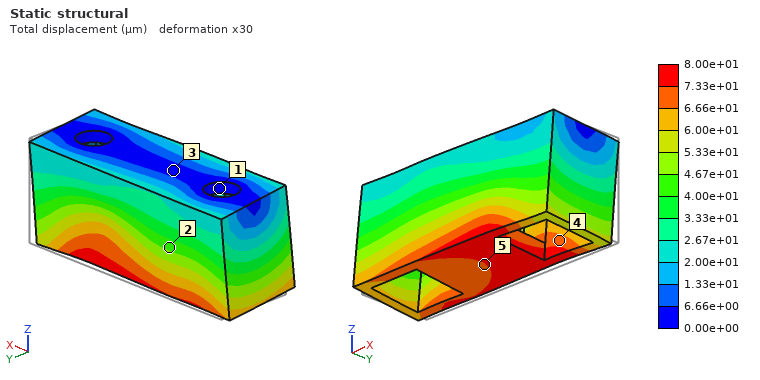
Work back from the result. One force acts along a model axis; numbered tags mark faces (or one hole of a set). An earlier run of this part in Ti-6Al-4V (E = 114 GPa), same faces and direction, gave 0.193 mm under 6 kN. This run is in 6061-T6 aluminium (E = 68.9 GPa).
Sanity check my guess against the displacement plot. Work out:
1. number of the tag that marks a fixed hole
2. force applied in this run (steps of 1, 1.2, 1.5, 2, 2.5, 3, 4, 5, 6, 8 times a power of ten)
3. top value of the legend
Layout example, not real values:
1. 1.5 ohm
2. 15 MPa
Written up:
1. 1
2. 1.5 kN
3. 8.00e+01 µm
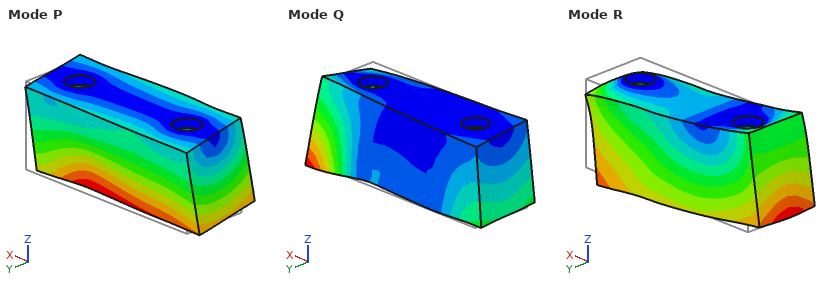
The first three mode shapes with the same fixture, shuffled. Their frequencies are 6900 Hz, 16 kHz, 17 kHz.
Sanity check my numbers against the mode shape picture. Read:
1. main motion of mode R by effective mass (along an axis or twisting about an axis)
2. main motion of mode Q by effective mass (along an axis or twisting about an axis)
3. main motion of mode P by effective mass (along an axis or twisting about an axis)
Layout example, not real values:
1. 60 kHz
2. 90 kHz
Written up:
1. along X
2. twisting about Z
3. along Y
